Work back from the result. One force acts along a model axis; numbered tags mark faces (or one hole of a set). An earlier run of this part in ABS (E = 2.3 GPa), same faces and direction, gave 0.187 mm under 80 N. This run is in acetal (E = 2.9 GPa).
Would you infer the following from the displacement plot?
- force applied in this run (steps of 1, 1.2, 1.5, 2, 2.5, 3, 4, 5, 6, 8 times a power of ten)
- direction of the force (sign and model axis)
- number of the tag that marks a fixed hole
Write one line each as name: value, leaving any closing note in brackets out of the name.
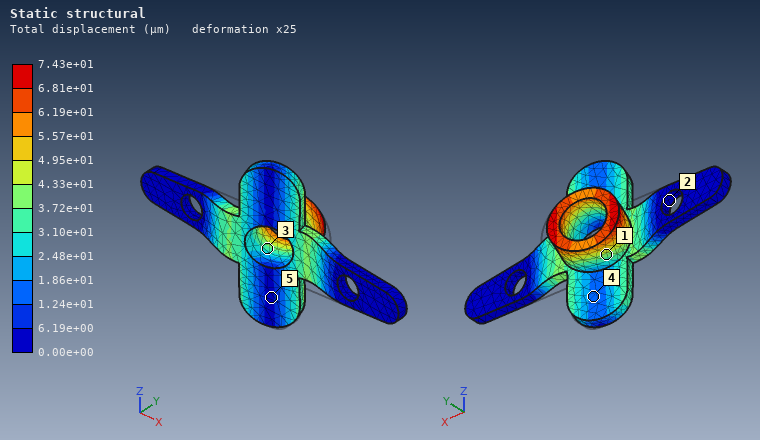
force applied in this run: 40 N
direction of the force: -X
number of the tag that marks a fixed hole: 2
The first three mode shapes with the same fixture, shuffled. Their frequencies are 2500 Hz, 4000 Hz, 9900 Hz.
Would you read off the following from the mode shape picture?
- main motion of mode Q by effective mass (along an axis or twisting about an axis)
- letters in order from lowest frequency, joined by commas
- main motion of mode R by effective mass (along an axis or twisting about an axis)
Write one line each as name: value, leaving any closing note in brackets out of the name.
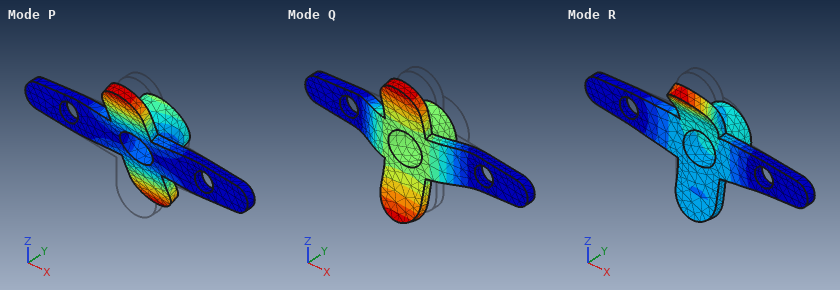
main motion of mode Q by effective mass: along Y
letters in order from lowest frequency, joined by commas: P, Q, R
main motion of mode R by effective mass: along Z
